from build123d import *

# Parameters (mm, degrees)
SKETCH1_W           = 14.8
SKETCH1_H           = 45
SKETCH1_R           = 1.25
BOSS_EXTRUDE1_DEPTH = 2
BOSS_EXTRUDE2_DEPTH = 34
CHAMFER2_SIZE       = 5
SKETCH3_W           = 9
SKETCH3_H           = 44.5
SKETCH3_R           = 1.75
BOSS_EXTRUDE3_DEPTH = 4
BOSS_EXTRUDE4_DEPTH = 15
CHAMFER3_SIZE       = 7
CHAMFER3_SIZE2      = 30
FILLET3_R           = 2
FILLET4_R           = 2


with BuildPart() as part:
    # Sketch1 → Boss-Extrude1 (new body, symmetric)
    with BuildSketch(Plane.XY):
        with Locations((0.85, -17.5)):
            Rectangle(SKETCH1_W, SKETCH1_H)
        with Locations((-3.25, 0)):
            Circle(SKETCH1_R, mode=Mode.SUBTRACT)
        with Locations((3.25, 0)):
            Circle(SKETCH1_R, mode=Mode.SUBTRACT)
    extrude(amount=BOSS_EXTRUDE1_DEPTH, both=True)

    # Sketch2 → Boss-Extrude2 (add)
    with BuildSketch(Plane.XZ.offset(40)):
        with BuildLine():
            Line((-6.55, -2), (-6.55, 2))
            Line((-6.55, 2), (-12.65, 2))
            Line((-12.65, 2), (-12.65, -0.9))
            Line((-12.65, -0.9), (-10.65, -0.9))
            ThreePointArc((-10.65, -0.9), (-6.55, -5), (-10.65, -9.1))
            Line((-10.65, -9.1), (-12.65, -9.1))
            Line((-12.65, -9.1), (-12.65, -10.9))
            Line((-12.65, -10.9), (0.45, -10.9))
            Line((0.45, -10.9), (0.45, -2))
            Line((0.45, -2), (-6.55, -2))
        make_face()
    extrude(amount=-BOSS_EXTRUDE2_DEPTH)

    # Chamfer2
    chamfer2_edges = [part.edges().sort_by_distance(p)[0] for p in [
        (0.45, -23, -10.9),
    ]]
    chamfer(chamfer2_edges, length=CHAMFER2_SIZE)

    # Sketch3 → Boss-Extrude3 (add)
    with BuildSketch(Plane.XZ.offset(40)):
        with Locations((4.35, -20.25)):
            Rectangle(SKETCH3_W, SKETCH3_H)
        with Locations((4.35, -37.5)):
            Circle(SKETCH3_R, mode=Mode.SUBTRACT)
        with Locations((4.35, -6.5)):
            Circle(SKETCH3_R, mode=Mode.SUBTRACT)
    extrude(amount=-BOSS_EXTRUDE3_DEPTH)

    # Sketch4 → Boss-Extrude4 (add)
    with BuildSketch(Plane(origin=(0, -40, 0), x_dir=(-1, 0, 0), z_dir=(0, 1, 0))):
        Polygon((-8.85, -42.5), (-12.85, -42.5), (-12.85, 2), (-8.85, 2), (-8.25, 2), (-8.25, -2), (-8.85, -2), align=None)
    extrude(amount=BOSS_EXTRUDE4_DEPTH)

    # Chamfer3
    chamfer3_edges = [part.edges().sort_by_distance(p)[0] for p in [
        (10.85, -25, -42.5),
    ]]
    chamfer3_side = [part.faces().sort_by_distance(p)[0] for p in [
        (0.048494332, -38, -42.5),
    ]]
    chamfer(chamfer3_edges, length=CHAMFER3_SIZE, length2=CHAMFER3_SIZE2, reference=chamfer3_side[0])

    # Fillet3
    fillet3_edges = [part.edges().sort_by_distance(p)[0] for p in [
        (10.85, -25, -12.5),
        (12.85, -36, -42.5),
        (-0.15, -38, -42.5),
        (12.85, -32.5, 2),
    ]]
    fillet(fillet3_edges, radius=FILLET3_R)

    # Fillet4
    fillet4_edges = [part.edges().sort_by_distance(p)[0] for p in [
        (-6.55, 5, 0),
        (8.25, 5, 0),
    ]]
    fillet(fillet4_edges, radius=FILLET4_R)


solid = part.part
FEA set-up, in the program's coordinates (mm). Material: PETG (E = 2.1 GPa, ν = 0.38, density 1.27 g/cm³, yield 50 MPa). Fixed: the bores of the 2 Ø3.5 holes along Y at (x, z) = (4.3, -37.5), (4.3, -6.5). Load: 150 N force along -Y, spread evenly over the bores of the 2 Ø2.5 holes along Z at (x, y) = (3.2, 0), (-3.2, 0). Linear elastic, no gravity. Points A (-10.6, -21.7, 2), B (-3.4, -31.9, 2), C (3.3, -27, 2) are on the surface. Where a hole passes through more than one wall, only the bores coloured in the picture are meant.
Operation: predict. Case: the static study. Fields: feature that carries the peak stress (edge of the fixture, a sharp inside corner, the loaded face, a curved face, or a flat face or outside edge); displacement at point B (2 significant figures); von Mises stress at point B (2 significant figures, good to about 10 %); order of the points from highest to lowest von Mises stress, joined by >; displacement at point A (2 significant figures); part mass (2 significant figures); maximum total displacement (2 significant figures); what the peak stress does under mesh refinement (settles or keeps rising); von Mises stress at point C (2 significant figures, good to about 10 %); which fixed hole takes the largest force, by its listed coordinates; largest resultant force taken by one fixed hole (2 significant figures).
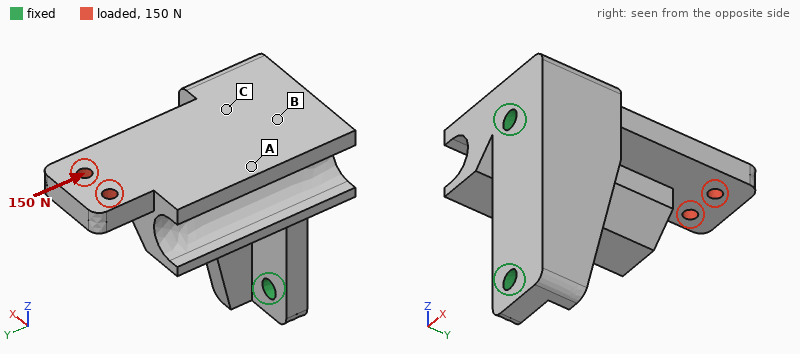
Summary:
edge of the fixture
0.17 mm
2.7 MPa
C > B > A
0.33 mm
12 g
0.63 mm
keeps rising
4.3 MPa
(4.3, -6.5)
170 N
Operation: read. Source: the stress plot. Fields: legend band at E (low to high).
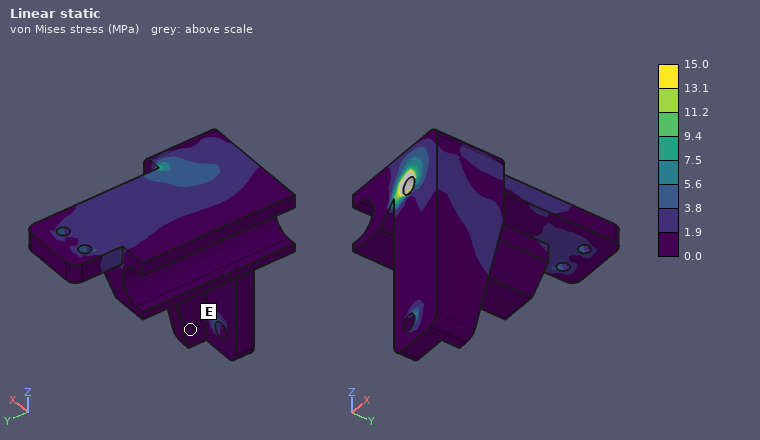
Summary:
0.0 to 1.9 MPa
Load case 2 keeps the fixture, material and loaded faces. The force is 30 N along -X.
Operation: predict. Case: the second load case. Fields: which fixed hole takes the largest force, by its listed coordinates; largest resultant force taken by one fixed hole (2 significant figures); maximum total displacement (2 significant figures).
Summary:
(4.3, -6.5)
34 N
0.78 mm
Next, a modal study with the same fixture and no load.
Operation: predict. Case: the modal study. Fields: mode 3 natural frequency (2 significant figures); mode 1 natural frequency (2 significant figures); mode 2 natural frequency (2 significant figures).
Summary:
2100 Hz
630 Hz
740 Hz
